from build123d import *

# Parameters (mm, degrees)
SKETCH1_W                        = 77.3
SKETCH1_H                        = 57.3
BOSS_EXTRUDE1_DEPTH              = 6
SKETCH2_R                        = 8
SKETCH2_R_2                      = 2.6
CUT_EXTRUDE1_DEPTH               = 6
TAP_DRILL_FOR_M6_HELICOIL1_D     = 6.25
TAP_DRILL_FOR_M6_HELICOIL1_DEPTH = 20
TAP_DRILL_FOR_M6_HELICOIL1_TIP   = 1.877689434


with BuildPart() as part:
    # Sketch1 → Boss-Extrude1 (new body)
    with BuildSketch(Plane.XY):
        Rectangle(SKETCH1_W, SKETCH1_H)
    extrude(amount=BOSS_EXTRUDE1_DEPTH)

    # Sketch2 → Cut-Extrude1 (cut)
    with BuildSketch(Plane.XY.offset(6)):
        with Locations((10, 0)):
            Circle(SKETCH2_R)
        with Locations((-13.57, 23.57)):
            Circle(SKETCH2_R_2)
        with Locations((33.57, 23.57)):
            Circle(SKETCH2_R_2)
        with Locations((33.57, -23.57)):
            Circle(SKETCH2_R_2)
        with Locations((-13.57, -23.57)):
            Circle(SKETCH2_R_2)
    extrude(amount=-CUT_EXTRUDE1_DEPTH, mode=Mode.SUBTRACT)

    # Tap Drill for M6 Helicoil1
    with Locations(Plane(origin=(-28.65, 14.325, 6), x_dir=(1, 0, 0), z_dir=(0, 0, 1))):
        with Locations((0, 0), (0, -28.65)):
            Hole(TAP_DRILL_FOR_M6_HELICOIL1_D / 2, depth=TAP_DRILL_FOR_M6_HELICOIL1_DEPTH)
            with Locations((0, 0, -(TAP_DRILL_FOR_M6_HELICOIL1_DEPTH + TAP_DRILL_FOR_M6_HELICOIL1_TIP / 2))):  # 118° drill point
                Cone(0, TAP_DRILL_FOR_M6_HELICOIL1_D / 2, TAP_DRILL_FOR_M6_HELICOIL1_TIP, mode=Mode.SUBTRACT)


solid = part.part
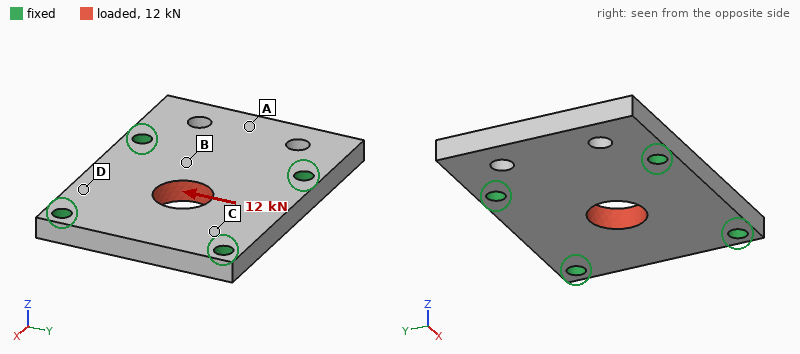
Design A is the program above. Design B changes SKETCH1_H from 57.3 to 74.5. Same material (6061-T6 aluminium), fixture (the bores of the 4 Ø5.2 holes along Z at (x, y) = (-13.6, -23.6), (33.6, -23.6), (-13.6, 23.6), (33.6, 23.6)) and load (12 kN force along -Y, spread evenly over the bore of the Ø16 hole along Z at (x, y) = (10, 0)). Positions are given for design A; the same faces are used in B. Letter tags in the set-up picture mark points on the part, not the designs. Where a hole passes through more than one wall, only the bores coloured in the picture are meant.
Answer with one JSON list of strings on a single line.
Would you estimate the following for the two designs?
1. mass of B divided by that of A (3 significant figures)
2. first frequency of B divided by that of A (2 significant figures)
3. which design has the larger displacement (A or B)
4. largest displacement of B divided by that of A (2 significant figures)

["1.33", "1.0", "A", "0.85"]
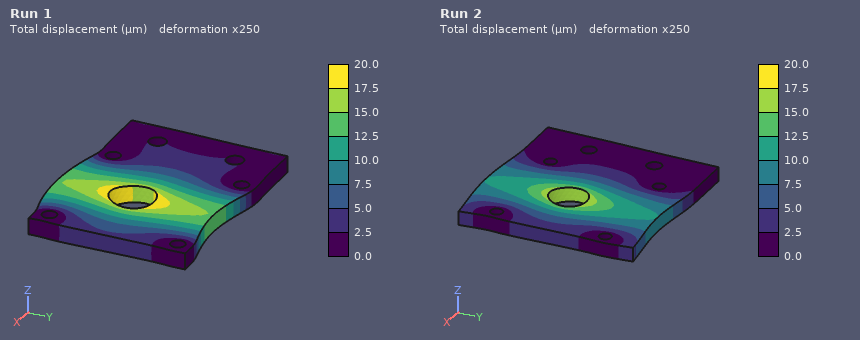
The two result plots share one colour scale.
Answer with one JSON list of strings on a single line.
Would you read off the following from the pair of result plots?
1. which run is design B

["Run 2"]
